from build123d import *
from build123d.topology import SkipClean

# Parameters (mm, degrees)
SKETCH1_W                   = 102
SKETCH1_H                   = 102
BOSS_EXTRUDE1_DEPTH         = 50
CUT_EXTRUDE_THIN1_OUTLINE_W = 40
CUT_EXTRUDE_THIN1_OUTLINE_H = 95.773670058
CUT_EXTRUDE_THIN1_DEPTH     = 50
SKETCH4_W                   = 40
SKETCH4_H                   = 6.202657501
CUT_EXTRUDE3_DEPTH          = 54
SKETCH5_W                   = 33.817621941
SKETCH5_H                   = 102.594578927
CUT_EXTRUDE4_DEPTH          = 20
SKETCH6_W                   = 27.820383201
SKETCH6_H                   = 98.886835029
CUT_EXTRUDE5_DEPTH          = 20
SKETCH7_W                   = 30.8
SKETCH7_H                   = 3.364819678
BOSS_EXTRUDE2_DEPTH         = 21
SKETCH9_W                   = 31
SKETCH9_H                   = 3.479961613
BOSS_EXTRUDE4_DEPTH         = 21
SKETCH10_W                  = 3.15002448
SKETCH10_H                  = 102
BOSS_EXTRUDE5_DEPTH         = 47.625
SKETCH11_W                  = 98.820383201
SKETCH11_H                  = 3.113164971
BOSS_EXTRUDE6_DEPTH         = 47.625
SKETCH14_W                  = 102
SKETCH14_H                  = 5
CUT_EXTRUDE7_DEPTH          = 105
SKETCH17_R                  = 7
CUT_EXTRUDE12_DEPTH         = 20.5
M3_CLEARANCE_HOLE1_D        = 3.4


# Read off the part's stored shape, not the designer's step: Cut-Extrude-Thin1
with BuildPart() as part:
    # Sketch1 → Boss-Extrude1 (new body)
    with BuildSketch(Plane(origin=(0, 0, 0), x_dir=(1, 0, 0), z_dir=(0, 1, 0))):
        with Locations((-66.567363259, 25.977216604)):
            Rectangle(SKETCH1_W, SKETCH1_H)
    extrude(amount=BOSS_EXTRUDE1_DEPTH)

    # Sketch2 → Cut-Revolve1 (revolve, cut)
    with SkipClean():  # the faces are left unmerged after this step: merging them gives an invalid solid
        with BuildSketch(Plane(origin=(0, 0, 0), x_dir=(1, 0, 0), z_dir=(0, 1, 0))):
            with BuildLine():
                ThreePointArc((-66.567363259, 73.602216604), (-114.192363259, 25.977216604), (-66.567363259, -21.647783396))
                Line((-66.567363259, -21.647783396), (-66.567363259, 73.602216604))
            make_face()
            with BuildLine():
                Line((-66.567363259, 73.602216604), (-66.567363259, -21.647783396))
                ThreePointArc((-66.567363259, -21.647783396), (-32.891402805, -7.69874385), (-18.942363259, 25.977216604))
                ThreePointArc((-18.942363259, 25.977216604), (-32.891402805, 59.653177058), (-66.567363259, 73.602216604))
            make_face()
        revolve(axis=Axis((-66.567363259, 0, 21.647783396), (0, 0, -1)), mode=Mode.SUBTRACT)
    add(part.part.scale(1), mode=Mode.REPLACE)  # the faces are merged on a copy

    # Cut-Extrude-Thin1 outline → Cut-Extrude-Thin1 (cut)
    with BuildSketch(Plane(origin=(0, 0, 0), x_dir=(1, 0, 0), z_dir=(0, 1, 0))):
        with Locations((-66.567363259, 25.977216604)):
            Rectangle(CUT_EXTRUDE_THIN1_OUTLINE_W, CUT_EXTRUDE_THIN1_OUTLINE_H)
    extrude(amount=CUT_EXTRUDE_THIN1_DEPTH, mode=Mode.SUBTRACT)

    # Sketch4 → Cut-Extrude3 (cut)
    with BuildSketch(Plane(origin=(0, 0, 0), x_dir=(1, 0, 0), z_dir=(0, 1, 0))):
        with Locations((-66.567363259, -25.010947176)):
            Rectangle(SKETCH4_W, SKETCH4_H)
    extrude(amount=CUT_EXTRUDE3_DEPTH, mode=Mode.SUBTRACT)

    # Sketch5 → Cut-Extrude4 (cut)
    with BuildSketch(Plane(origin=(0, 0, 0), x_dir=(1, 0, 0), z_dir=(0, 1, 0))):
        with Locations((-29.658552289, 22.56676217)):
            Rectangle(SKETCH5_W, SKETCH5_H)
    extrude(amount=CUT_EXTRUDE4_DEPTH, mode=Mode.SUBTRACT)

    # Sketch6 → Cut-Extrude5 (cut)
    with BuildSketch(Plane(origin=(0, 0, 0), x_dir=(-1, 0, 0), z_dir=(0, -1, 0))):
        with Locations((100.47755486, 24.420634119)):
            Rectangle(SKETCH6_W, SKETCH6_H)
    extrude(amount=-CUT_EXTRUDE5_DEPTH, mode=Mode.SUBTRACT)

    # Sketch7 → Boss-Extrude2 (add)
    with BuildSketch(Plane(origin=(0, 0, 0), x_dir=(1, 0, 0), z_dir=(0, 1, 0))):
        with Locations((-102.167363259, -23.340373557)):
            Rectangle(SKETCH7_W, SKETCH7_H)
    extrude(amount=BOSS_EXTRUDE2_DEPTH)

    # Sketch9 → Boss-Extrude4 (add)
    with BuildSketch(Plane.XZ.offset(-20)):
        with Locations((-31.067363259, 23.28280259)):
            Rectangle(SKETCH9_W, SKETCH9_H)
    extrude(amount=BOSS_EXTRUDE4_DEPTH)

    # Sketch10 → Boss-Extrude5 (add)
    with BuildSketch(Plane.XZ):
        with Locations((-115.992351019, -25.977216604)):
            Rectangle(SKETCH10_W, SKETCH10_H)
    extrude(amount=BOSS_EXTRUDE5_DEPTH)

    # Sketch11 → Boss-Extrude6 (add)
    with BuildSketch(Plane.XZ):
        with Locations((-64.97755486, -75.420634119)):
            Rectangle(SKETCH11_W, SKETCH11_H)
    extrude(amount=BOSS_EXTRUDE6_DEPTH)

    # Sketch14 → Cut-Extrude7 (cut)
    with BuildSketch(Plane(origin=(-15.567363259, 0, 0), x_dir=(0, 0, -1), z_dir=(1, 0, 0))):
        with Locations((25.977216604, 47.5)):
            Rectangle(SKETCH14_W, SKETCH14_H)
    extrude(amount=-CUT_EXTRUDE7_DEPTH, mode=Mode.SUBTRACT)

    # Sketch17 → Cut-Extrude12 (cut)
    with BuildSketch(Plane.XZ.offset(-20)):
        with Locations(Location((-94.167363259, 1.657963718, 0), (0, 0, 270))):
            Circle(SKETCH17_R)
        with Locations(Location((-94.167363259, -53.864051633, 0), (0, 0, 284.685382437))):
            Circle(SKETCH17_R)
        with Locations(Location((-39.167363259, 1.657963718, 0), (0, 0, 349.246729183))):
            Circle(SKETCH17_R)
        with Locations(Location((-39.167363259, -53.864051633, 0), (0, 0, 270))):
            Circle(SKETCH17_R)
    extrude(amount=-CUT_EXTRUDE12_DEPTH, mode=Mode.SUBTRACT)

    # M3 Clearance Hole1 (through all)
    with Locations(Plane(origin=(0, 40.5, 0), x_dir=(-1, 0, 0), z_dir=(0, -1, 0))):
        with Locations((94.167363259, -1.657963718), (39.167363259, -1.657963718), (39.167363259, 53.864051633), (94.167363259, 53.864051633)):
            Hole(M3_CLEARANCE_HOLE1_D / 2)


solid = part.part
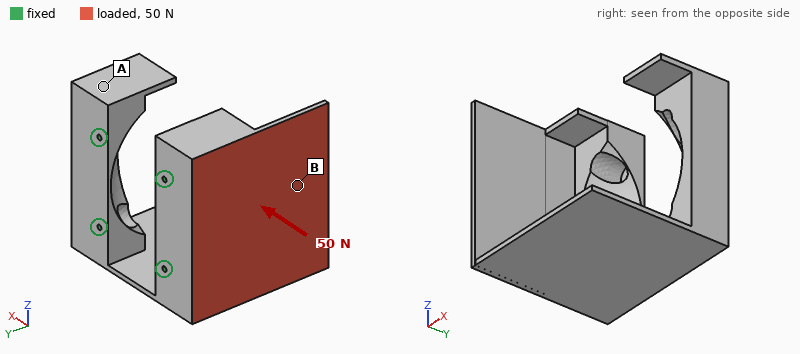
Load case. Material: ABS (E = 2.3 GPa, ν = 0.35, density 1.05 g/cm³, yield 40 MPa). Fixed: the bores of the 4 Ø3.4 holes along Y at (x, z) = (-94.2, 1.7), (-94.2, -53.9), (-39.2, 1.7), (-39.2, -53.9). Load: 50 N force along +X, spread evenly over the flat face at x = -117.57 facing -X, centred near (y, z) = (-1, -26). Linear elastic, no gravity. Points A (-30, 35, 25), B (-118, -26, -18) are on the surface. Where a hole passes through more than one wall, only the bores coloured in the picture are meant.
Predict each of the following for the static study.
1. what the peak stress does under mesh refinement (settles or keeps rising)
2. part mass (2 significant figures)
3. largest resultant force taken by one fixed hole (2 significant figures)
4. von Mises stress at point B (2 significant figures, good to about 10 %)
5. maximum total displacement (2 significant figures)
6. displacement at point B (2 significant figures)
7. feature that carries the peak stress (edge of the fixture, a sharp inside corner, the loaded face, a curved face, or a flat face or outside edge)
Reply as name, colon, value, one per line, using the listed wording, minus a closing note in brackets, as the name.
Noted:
what the peak stress does under mesh refinement: keeps rising
part mass: 180 g
largest resultant force taken by one fixed hole: 40 N
von Mises stress at point B: 1.2 MPa
maximum total displacement: 1.8 mm
displacement at point B: 1.1 mm
feature that carries the peak stress: a sharp inside corner
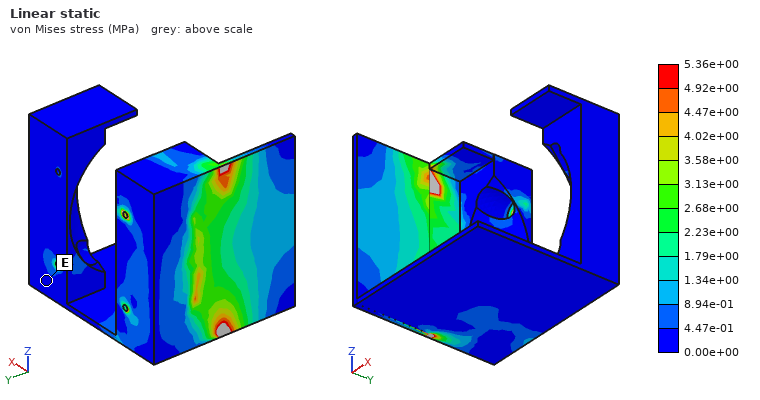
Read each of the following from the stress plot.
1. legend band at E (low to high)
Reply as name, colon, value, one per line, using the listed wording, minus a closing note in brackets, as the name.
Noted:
legend band at E: 0.00e+00 to 4.47e-01 MPa
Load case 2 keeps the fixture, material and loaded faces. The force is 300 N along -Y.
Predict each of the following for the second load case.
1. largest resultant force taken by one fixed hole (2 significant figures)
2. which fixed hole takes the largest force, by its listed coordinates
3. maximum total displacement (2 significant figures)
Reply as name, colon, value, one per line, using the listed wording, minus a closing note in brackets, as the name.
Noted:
largest resultant force taken by one fixed hole: 260 N
which fixed hole takes the largest force, by its listed coordinates: (-94.2, -53.9)
maximum total displacement: 1.5 mm
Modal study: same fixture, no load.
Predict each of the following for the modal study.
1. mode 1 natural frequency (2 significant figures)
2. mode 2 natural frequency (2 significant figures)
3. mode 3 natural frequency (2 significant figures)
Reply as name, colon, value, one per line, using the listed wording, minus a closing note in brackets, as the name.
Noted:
mode 1 natural frequency: 170 Hz
mode 2 natural frequency: 200 Hz
mode 3 natural frequency: 350 Hz
